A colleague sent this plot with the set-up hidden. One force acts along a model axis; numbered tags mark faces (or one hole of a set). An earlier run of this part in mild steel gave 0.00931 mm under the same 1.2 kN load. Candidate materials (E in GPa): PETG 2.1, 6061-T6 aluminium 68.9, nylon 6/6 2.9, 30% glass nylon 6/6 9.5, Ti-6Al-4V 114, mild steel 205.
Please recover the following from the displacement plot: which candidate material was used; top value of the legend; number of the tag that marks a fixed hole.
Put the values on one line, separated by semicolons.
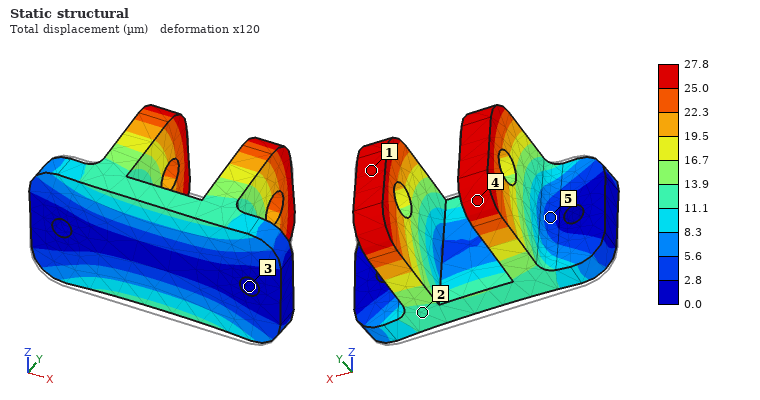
6061-T6 aluminium; 27.8 µm; 3
